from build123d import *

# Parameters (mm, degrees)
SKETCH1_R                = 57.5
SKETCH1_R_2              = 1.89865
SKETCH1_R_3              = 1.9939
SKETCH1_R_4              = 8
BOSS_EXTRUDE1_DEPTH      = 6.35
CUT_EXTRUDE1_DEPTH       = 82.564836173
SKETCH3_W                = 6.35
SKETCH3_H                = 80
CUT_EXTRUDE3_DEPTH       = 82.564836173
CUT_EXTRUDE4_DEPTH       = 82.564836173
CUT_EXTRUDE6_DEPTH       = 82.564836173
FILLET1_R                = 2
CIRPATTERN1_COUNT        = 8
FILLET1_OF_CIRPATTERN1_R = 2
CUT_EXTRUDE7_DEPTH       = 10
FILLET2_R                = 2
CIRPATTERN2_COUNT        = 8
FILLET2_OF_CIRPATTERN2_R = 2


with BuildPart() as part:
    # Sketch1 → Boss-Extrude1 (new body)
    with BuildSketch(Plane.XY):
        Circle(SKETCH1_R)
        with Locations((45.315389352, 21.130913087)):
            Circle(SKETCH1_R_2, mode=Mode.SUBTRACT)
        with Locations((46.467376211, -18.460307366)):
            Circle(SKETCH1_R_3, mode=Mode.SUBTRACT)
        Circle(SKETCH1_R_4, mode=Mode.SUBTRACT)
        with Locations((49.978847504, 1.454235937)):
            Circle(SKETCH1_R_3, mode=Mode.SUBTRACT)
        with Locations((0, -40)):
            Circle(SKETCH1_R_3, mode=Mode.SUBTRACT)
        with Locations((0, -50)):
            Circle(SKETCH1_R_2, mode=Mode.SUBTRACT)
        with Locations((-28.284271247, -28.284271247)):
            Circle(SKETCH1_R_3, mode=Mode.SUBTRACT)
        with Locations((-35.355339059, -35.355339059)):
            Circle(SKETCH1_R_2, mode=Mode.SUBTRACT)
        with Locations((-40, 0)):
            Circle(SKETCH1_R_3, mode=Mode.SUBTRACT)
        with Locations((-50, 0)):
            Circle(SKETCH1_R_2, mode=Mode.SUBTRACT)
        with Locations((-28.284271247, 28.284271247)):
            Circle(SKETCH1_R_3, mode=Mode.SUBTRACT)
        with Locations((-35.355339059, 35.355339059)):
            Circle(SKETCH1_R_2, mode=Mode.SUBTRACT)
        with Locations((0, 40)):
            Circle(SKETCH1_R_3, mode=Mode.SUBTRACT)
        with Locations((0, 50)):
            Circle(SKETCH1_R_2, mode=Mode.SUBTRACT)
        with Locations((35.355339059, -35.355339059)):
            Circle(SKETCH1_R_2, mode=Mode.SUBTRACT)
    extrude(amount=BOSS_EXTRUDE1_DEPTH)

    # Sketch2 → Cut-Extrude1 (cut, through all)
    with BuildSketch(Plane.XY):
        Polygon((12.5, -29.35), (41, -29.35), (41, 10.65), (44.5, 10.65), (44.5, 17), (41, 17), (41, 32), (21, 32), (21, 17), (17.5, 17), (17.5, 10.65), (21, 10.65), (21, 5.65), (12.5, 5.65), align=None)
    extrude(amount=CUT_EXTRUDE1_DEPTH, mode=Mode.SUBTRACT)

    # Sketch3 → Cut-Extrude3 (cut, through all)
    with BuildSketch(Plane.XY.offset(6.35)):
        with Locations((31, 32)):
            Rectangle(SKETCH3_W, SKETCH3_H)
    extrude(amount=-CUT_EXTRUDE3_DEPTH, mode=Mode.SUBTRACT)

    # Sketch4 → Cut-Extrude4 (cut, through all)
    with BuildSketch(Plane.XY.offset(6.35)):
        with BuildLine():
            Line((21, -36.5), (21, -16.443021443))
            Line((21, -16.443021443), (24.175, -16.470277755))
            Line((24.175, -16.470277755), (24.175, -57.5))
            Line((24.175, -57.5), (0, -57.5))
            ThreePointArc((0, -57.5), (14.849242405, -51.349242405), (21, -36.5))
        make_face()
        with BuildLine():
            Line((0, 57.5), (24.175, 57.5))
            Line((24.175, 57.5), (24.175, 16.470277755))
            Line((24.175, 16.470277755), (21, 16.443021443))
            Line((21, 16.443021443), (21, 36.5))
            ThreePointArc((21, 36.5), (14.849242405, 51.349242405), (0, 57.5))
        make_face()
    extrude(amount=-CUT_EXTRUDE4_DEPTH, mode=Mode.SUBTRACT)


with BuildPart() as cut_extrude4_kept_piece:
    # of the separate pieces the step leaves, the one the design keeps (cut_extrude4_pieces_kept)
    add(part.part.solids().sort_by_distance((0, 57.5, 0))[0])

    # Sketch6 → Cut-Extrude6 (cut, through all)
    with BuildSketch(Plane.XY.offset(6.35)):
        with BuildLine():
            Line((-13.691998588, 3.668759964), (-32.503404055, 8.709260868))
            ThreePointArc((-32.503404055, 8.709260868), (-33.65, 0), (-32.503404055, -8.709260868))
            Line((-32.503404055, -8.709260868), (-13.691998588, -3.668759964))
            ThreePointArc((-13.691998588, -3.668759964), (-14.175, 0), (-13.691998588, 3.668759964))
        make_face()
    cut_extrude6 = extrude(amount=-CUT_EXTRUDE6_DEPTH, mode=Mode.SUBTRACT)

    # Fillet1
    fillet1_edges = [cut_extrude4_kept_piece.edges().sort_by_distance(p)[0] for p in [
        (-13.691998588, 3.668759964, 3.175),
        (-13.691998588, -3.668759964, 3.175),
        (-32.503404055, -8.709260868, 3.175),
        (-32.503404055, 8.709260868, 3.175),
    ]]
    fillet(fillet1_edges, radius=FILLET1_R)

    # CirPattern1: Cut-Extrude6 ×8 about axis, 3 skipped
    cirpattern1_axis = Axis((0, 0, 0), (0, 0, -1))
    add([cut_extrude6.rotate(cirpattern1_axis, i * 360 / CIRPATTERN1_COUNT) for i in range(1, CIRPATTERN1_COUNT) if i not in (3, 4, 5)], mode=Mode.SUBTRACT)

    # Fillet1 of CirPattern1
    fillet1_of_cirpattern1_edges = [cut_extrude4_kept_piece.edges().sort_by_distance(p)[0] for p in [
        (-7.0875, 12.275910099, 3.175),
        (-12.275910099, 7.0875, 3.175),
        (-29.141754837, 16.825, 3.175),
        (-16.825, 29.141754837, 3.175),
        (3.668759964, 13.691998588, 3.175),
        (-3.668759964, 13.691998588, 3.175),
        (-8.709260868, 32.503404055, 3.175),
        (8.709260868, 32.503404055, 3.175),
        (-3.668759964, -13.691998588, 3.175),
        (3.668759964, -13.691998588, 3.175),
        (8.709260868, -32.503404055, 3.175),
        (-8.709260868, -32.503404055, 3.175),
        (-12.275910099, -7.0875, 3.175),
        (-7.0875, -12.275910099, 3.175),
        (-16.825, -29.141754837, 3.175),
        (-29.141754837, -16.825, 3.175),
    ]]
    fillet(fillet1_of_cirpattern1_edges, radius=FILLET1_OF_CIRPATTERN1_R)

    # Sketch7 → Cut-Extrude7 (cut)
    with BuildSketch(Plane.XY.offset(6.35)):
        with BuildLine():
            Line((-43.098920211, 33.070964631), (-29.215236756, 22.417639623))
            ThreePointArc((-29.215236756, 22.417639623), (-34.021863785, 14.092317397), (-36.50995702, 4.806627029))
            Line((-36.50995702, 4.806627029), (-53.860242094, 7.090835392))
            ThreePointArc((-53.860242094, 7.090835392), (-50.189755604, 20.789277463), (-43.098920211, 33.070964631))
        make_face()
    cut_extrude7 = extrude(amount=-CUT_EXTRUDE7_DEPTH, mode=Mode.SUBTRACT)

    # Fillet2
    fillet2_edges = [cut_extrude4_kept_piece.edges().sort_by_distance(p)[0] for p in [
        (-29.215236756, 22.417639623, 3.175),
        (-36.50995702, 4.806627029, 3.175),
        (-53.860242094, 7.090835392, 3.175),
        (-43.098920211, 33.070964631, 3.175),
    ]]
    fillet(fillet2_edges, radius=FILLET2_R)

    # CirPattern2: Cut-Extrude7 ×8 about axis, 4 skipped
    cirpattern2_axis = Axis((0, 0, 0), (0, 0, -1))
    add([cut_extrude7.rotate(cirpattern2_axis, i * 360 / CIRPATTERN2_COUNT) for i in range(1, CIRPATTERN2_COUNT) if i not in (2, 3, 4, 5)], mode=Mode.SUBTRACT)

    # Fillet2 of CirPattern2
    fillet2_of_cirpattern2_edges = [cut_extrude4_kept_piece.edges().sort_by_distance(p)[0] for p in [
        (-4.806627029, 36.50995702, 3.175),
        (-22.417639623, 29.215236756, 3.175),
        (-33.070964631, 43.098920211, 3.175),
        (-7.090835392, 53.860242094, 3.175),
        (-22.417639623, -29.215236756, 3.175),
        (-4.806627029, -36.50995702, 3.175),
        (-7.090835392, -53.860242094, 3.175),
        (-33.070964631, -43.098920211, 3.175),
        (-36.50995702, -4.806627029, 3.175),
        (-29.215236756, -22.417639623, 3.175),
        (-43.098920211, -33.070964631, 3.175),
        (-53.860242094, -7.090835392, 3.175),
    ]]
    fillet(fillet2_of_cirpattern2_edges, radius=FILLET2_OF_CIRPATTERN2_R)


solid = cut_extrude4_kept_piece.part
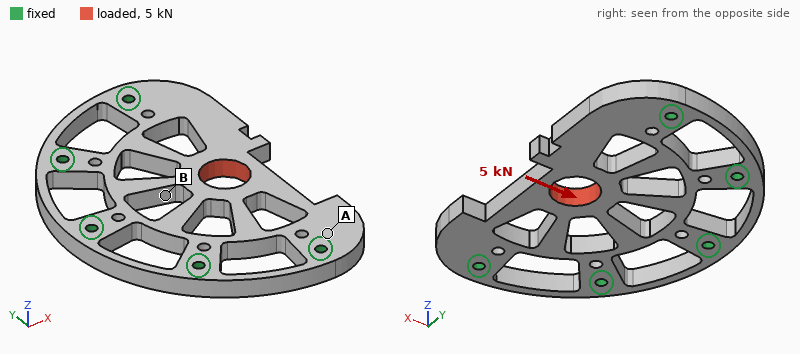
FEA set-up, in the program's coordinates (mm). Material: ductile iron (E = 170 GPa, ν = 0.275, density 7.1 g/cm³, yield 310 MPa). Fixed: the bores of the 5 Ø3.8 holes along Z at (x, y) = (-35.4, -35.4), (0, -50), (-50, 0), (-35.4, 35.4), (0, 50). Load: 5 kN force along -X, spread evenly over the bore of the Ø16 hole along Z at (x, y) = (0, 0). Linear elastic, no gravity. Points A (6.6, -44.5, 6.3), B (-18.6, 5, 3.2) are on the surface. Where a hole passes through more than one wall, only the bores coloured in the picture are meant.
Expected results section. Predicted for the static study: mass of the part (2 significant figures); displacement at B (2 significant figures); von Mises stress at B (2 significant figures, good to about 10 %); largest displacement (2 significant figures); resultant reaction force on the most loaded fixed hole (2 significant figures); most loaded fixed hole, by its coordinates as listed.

180 g
19 µm
40 MPa
31 µm
2.0 kN
(-50, 0)
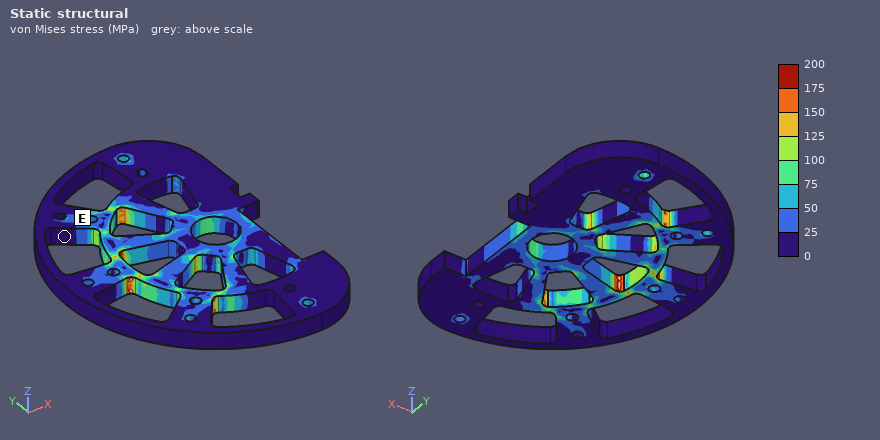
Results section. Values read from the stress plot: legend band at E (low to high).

0 to 25 MPa
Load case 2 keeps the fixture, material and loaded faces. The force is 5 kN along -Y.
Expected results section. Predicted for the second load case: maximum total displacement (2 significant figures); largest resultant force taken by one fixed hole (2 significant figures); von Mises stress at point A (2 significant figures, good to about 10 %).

14 µm
1.8 kN
17 MPa
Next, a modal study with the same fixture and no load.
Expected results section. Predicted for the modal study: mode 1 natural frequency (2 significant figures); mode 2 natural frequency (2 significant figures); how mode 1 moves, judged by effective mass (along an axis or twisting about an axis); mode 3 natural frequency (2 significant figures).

3000 Hz
6300 Hz
along Z
7400 Hz
